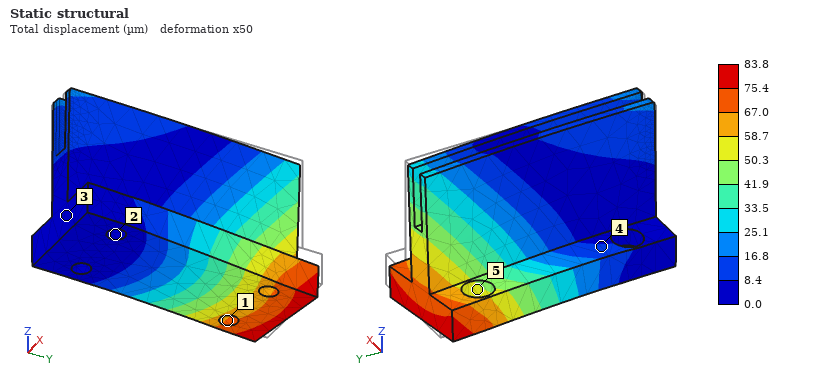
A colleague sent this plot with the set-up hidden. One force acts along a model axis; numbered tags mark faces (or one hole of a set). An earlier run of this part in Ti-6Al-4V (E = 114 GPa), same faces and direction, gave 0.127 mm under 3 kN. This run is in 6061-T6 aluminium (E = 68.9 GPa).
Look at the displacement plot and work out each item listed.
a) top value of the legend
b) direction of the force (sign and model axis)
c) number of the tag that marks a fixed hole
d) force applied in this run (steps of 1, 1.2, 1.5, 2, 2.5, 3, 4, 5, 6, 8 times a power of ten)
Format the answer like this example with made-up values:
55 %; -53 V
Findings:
83.8 µm; -X; 2; 1.2 kN
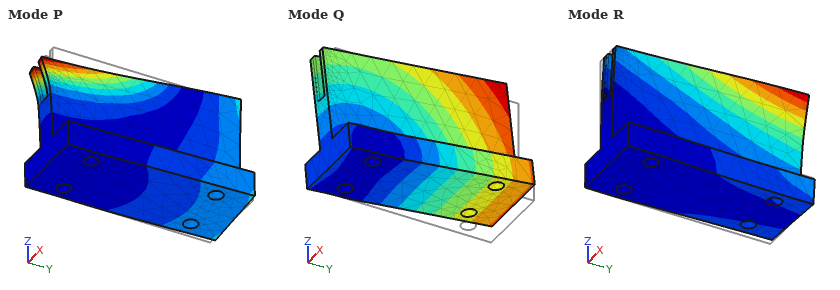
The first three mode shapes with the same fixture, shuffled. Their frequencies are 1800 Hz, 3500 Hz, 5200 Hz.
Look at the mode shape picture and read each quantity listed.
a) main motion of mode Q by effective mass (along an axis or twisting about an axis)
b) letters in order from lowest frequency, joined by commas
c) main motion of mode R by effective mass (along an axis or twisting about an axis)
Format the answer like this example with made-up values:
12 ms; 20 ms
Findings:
along Z; Q, R, P; along X
